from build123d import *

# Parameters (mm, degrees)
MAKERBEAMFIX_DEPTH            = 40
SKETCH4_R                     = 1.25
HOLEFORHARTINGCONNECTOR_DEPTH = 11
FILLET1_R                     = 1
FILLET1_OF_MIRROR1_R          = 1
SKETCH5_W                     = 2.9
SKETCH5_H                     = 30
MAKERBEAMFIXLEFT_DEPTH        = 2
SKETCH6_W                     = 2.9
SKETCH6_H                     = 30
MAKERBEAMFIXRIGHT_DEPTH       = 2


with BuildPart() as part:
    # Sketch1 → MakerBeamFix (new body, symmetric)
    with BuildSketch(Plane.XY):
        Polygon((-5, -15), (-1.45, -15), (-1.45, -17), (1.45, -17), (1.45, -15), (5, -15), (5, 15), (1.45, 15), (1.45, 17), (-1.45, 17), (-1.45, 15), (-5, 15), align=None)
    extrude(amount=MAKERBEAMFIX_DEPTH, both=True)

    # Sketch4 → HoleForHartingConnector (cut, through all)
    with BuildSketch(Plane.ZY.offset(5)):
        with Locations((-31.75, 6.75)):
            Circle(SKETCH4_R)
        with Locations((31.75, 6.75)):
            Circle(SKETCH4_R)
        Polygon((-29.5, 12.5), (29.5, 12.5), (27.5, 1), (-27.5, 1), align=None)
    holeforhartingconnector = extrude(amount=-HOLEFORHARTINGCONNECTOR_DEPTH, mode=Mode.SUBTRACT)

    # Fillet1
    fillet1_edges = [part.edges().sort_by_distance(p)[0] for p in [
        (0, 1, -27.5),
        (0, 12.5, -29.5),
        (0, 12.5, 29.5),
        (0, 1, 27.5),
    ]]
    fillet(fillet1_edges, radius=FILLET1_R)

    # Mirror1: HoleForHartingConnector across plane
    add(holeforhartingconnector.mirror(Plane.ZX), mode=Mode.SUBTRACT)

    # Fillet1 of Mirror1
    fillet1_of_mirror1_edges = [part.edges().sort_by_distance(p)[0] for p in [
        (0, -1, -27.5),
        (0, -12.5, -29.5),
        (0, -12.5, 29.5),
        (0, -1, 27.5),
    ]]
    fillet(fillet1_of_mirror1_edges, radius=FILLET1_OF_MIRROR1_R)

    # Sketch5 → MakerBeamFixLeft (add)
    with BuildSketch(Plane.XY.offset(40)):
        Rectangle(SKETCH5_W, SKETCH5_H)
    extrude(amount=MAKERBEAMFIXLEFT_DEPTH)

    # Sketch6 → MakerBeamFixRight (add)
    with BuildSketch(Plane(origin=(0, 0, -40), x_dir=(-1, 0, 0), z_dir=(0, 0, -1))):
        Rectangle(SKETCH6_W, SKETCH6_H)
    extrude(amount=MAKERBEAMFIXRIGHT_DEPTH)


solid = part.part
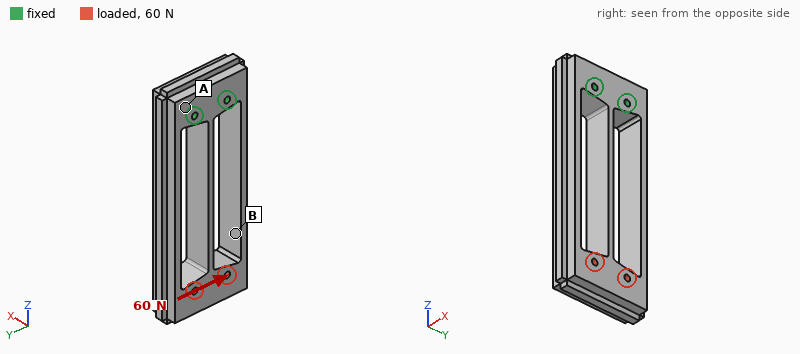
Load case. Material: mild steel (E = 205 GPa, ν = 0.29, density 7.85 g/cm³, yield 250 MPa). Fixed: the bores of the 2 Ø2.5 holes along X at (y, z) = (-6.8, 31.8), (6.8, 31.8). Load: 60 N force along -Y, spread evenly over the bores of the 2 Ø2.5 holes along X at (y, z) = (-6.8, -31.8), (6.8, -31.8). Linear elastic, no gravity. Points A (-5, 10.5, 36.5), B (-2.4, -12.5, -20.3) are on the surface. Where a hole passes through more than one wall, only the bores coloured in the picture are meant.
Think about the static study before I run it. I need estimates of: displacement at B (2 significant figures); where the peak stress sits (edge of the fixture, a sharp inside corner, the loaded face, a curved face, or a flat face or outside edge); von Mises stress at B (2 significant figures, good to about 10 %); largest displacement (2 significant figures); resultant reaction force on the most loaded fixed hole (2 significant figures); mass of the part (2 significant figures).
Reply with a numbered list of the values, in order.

1. 67 µm
2. a curved face
3. 26 MPa
4. 75 µm
5. 230 N
6. 94 g
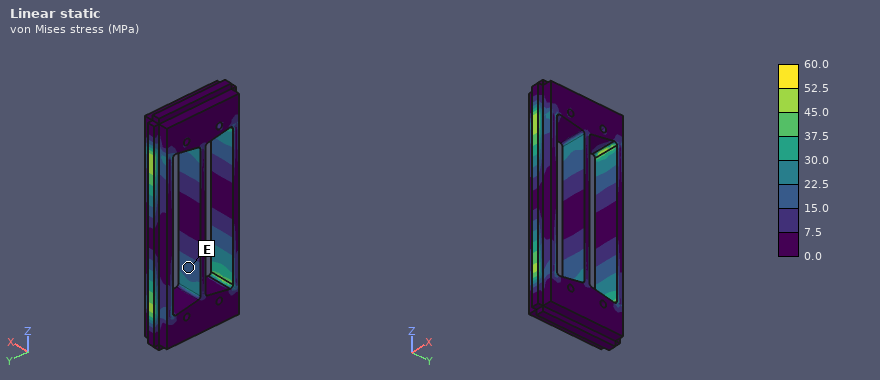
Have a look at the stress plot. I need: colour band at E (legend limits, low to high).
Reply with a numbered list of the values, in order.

1. 15.0 to 22.5 MPa
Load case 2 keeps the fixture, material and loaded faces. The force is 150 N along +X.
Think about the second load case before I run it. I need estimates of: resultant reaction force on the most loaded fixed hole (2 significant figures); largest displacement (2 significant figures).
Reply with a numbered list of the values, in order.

1. 75 N
2. 0.14 mm
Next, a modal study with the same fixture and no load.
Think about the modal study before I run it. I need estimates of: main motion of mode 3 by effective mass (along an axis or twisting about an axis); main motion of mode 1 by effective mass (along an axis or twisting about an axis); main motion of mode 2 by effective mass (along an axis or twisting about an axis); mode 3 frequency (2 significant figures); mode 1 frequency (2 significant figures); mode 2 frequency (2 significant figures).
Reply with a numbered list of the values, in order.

1. twisting about Z
2. along Y
3. along X
4. 2100 Hz
5. 700 Hz
6. 900 Hz
